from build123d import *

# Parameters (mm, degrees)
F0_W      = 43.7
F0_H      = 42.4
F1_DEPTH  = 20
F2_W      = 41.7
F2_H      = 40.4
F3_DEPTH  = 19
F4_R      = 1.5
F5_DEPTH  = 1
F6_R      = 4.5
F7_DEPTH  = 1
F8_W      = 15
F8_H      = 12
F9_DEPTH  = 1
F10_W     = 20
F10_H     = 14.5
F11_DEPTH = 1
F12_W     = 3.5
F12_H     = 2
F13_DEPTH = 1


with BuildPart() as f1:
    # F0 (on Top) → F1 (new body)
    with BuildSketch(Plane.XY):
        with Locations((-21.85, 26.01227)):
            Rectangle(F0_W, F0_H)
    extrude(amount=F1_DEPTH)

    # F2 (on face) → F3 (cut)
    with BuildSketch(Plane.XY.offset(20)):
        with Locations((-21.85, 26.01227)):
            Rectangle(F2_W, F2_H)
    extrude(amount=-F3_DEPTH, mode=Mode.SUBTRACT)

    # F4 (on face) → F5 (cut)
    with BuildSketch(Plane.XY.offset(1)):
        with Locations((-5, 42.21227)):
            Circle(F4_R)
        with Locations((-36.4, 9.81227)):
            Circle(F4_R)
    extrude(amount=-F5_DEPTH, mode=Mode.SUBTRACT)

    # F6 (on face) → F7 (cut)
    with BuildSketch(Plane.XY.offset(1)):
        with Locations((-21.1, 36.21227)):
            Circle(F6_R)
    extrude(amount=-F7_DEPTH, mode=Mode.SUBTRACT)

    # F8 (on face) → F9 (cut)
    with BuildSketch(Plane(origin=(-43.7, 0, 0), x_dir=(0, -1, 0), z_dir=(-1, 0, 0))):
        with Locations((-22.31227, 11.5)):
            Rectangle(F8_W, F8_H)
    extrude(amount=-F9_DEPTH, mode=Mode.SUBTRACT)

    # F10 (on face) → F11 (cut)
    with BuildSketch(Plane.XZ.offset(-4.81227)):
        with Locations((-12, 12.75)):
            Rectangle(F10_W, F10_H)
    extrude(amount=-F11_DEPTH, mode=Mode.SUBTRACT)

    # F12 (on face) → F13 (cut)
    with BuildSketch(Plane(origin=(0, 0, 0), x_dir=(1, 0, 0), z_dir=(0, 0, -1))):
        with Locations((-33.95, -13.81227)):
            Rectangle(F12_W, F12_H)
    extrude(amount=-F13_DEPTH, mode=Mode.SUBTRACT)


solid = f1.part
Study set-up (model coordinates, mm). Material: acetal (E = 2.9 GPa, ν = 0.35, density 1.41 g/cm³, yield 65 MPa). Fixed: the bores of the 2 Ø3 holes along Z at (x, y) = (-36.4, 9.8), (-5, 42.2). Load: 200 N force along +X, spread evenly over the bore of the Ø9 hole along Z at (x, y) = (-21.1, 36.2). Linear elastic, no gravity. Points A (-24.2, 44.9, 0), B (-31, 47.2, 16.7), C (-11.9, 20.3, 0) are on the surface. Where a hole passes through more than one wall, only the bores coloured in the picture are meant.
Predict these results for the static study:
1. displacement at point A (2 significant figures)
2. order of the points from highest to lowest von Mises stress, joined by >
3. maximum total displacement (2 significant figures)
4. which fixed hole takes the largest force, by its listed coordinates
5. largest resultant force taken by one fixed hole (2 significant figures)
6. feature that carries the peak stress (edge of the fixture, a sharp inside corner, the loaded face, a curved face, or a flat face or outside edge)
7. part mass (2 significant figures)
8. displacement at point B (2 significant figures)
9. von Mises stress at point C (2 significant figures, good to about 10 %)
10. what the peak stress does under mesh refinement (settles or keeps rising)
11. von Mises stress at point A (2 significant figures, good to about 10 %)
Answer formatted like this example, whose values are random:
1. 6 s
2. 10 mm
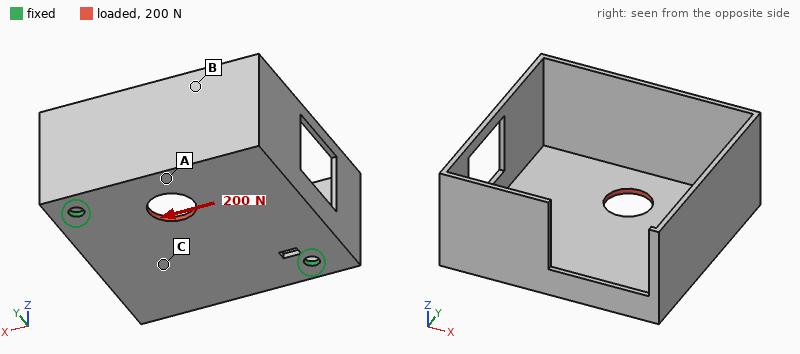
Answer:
1. 58 µm
2. A > C > B
3. 83 µm
4. (-5, 42.2)
5. 150 N
6. edge of the fixture
7. 6.3 g
8. 46 µm
9. 2.7 MPa
10. keeps rising
11. 4.2 MPa
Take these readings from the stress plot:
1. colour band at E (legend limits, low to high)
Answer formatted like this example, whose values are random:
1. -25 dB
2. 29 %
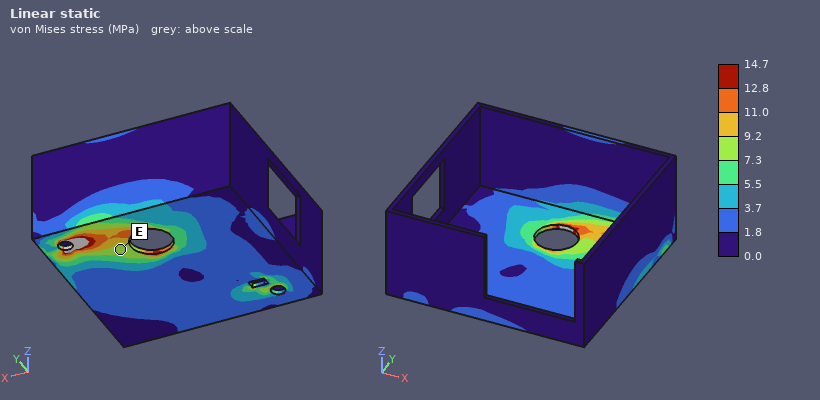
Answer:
1. 7.3 to 9.2 MPa
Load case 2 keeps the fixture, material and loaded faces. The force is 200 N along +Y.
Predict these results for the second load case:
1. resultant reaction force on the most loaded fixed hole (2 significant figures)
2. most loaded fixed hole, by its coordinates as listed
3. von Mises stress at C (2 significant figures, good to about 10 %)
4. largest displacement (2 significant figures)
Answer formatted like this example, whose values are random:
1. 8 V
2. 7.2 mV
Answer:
1. 110 N
2. (-5, 42.2)
3. 3.1 MPa
4. 0.10 mm
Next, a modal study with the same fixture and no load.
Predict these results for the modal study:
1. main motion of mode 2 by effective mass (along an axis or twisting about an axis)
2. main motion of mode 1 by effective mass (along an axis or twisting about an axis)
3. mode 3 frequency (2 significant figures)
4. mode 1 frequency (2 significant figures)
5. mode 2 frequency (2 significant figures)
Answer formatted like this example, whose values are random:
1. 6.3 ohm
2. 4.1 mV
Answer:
1. along Z
2. along Z
3. 760 Hz
4. 290 Hz
5. 370 Hz
